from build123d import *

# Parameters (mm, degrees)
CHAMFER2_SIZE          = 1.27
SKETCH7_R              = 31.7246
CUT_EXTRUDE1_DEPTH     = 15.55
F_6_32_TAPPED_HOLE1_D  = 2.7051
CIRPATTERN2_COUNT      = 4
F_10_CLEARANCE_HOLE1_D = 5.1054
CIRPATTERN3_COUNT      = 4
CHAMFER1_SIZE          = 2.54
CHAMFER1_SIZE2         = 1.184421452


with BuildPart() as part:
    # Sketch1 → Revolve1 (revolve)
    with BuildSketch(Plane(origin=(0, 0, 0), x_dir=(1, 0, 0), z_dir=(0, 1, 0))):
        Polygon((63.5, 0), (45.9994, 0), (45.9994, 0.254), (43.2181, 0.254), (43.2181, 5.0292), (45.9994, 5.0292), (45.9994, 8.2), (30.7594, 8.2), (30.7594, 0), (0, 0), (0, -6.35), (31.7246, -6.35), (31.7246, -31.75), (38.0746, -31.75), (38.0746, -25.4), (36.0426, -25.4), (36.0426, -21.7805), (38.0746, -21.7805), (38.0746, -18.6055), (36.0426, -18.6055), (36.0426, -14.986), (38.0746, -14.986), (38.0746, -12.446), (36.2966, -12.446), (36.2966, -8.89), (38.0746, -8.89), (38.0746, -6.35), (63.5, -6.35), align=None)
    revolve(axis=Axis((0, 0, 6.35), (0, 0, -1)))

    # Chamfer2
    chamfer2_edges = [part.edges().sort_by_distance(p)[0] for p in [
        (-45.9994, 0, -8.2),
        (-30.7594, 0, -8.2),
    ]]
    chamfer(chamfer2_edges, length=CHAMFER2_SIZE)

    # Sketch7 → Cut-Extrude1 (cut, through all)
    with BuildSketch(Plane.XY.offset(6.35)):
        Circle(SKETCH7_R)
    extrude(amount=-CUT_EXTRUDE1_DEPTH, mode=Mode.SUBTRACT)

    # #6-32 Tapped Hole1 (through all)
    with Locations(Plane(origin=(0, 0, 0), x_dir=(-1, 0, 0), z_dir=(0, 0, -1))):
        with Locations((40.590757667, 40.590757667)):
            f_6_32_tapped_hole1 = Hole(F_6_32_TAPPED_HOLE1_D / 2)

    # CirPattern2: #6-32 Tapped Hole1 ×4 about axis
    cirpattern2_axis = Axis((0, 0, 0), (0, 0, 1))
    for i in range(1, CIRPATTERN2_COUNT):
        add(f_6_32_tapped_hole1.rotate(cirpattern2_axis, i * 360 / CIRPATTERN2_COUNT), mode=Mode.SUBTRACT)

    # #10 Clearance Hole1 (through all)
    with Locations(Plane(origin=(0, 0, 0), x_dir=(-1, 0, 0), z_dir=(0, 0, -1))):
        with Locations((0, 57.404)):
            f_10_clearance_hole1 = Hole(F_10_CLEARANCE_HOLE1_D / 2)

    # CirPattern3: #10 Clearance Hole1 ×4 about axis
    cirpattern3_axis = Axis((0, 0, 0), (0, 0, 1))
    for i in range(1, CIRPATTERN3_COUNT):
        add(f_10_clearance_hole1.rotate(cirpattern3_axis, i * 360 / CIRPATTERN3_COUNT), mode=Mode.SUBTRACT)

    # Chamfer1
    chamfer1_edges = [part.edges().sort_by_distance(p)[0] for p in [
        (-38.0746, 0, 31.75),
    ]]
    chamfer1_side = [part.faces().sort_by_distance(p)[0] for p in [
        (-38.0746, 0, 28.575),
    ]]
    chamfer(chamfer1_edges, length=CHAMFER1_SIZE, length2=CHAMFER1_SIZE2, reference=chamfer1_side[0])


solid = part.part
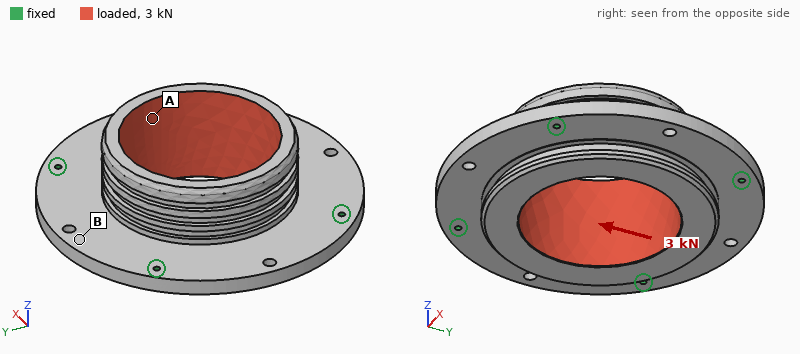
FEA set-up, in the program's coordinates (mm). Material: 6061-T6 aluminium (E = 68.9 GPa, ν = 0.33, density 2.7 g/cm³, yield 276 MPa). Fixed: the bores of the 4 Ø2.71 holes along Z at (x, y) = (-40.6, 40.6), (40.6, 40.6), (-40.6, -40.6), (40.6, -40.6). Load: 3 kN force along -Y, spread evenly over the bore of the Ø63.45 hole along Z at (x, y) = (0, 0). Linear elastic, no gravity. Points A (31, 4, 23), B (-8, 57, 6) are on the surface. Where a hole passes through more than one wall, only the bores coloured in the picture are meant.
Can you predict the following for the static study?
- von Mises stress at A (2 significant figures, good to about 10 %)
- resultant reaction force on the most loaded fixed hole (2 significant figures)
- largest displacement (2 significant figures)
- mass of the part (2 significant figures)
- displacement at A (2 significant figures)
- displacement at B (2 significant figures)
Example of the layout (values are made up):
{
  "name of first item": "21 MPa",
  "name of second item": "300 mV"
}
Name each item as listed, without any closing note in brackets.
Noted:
{
  "von Mises stress at A": "3.5 MPa",
  "resultant reaction force on the most loaded fixed hole": "770 N",
  "largest displacement": "13 µm",
  "mass of the part": "310 g",
  "displacement at A": "6.6 µm",
  "displacement at B": "8.4 µm"
}
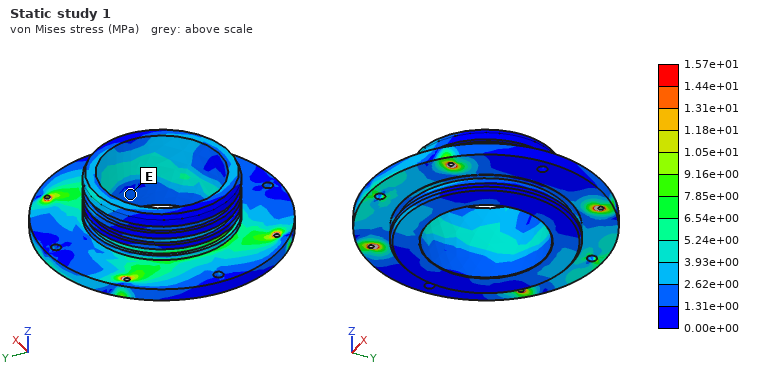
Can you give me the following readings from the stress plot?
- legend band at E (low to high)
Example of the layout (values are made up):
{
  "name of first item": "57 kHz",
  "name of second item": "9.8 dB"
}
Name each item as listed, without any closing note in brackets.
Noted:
{
  "legend band at E": "1.31e+00 to 2.62e+00 MPa"
}
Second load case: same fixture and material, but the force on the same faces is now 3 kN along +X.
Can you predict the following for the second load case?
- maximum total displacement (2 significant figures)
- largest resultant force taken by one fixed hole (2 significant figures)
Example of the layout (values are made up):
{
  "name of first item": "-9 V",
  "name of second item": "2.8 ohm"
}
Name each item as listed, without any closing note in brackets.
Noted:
{
  "maximum total displacement": "13 µm",
  "largest resultant force taken by one fixed hole": "770 N"
}
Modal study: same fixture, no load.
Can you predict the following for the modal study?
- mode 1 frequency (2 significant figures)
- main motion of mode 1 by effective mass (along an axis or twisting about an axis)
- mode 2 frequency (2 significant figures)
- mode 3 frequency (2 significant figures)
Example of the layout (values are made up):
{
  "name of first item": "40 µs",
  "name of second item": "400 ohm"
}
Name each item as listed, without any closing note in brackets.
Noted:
{
  "mode 1 frequency": "3800 Hz",
  "main motion of mode 1 by effective mass": "along Z",
  "mode 2 frequency": "4200 Hz",
  "mode 3 frequency": "4300 Hz"
}
